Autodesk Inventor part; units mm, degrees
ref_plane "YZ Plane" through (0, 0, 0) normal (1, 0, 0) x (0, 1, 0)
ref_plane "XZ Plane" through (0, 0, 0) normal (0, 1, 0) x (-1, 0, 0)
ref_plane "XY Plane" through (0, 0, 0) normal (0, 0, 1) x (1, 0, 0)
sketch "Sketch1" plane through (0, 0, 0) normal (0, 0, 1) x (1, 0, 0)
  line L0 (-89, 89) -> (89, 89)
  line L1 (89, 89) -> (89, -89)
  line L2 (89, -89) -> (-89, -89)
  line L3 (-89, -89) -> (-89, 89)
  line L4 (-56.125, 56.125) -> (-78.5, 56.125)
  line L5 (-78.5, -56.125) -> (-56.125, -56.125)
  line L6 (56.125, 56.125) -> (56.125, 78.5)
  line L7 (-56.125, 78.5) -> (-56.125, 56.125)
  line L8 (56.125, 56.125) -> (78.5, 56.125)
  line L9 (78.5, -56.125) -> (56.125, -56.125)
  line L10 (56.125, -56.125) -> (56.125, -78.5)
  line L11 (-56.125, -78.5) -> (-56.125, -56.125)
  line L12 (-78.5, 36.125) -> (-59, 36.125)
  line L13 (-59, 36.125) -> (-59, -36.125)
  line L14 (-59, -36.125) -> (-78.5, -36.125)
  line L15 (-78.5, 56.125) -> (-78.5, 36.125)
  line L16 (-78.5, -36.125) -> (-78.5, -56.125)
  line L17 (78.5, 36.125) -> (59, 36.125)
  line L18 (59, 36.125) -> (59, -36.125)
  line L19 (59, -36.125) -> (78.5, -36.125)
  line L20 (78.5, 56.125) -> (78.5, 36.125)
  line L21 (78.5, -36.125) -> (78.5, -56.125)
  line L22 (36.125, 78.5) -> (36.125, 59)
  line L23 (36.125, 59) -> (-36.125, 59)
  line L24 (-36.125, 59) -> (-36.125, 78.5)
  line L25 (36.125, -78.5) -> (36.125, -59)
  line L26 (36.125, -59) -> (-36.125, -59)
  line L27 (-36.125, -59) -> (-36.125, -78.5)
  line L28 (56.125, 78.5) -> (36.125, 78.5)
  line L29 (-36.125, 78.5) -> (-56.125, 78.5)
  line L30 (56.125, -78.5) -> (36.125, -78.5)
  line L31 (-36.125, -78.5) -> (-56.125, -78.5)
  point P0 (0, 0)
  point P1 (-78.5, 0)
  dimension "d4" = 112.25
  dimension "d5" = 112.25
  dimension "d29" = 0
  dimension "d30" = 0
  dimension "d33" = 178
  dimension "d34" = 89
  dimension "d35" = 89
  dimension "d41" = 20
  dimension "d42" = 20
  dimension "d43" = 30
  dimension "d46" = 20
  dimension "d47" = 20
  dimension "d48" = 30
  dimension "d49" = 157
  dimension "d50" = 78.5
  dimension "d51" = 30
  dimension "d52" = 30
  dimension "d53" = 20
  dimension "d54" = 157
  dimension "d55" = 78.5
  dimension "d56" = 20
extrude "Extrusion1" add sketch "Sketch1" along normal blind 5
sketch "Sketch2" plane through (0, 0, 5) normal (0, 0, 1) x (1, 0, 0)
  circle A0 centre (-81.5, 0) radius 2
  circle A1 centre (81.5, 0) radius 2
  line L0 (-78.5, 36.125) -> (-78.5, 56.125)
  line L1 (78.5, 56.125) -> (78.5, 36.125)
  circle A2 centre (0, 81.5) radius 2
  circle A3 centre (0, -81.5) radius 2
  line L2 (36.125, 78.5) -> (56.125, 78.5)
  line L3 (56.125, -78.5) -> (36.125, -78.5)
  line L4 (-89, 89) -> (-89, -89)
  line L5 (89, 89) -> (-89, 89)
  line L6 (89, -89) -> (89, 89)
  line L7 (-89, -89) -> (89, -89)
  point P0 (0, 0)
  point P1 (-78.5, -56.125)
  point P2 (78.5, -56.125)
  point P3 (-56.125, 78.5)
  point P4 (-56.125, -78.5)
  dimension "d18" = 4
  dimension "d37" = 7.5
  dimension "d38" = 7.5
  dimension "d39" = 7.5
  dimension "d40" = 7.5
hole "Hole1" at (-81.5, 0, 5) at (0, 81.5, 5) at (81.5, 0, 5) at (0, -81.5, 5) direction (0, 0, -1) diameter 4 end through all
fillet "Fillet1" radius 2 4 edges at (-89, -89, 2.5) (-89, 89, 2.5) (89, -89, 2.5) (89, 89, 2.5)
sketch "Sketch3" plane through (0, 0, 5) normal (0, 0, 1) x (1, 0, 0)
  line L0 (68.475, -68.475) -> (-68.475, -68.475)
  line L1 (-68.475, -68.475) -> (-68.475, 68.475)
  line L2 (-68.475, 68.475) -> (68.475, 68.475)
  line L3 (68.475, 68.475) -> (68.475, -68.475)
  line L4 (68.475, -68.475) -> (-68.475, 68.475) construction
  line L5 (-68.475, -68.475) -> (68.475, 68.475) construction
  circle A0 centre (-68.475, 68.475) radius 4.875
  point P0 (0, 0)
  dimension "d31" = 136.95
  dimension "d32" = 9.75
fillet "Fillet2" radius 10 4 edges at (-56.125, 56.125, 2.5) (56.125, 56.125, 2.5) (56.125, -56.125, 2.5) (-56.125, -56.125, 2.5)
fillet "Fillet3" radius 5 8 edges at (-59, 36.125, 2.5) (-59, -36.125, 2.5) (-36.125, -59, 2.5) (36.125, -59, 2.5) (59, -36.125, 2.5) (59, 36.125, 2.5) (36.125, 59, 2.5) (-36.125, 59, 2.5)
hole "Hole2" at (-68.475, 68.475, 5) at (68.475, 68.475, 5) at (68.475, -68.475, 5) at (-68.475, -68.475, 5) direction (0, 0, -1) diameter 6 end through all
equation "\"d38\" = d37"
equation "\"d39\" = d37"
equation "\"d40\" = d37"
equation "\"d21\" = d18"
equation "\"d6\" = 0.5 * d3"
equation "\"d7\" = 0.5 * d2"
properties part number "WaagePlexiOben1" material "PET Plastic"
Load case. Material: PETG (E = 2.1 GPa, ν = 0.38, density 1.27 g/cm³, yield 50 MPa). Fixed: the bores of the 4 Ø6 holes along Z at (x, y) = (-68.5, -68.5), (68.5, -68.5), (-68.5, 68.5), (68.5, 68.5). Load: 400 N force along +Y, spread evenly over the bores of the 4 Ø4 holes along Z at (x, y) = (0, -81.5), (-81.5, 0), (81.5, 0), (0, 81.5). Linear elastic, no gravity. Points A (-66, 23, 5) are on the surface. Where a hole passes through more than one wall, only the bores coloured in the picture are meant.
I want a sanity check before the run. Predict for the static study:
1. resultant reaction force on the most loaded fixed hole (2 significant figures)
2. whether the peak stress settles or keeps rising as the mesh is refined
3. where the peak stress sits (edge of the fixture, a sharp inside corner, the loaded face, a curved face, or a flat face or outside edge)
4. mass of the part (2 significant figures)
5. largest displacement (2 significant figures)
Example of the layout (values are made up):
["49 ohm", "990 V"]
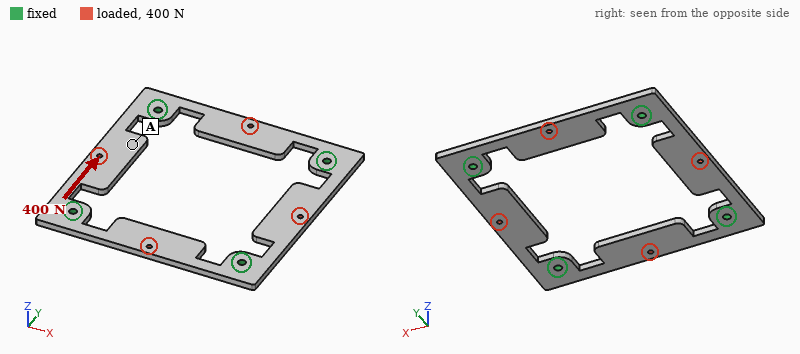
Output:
["100 N", "keeps rising", "a sharp inside corner", "91 g", "0.27 mm"]
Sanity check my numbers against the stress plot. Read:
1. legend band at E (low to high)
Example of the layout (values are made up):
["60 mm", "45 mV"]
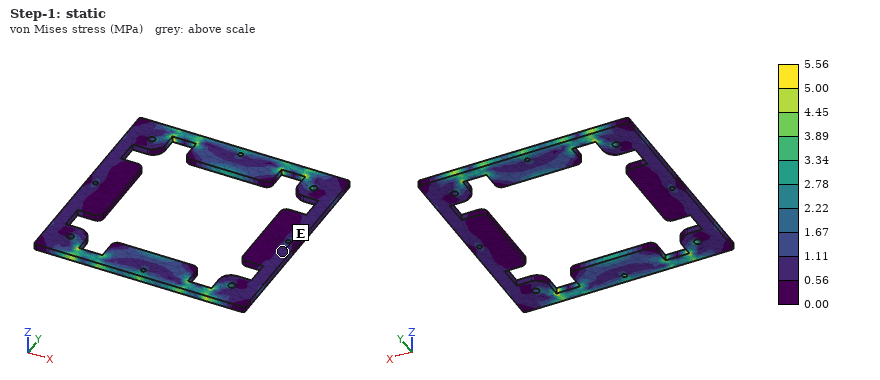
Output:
["0.56 to 1.11 MPa"]
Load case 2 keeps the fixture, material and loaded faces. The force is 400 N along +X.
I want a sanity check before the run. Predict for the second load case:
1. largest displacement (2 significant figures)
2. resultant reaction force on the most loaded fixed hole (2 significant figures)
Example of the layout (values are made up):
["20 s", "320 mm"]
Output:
["0.27 mm", "100 N"]
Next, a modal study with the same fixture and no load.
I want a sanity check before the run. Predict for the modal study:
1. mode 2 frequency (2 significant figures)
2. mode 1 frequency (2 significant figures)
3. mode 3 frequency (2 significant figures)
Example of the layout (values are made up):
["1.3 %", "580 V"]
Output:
["250 Hz", "250 Hz", "250 Hz"]
